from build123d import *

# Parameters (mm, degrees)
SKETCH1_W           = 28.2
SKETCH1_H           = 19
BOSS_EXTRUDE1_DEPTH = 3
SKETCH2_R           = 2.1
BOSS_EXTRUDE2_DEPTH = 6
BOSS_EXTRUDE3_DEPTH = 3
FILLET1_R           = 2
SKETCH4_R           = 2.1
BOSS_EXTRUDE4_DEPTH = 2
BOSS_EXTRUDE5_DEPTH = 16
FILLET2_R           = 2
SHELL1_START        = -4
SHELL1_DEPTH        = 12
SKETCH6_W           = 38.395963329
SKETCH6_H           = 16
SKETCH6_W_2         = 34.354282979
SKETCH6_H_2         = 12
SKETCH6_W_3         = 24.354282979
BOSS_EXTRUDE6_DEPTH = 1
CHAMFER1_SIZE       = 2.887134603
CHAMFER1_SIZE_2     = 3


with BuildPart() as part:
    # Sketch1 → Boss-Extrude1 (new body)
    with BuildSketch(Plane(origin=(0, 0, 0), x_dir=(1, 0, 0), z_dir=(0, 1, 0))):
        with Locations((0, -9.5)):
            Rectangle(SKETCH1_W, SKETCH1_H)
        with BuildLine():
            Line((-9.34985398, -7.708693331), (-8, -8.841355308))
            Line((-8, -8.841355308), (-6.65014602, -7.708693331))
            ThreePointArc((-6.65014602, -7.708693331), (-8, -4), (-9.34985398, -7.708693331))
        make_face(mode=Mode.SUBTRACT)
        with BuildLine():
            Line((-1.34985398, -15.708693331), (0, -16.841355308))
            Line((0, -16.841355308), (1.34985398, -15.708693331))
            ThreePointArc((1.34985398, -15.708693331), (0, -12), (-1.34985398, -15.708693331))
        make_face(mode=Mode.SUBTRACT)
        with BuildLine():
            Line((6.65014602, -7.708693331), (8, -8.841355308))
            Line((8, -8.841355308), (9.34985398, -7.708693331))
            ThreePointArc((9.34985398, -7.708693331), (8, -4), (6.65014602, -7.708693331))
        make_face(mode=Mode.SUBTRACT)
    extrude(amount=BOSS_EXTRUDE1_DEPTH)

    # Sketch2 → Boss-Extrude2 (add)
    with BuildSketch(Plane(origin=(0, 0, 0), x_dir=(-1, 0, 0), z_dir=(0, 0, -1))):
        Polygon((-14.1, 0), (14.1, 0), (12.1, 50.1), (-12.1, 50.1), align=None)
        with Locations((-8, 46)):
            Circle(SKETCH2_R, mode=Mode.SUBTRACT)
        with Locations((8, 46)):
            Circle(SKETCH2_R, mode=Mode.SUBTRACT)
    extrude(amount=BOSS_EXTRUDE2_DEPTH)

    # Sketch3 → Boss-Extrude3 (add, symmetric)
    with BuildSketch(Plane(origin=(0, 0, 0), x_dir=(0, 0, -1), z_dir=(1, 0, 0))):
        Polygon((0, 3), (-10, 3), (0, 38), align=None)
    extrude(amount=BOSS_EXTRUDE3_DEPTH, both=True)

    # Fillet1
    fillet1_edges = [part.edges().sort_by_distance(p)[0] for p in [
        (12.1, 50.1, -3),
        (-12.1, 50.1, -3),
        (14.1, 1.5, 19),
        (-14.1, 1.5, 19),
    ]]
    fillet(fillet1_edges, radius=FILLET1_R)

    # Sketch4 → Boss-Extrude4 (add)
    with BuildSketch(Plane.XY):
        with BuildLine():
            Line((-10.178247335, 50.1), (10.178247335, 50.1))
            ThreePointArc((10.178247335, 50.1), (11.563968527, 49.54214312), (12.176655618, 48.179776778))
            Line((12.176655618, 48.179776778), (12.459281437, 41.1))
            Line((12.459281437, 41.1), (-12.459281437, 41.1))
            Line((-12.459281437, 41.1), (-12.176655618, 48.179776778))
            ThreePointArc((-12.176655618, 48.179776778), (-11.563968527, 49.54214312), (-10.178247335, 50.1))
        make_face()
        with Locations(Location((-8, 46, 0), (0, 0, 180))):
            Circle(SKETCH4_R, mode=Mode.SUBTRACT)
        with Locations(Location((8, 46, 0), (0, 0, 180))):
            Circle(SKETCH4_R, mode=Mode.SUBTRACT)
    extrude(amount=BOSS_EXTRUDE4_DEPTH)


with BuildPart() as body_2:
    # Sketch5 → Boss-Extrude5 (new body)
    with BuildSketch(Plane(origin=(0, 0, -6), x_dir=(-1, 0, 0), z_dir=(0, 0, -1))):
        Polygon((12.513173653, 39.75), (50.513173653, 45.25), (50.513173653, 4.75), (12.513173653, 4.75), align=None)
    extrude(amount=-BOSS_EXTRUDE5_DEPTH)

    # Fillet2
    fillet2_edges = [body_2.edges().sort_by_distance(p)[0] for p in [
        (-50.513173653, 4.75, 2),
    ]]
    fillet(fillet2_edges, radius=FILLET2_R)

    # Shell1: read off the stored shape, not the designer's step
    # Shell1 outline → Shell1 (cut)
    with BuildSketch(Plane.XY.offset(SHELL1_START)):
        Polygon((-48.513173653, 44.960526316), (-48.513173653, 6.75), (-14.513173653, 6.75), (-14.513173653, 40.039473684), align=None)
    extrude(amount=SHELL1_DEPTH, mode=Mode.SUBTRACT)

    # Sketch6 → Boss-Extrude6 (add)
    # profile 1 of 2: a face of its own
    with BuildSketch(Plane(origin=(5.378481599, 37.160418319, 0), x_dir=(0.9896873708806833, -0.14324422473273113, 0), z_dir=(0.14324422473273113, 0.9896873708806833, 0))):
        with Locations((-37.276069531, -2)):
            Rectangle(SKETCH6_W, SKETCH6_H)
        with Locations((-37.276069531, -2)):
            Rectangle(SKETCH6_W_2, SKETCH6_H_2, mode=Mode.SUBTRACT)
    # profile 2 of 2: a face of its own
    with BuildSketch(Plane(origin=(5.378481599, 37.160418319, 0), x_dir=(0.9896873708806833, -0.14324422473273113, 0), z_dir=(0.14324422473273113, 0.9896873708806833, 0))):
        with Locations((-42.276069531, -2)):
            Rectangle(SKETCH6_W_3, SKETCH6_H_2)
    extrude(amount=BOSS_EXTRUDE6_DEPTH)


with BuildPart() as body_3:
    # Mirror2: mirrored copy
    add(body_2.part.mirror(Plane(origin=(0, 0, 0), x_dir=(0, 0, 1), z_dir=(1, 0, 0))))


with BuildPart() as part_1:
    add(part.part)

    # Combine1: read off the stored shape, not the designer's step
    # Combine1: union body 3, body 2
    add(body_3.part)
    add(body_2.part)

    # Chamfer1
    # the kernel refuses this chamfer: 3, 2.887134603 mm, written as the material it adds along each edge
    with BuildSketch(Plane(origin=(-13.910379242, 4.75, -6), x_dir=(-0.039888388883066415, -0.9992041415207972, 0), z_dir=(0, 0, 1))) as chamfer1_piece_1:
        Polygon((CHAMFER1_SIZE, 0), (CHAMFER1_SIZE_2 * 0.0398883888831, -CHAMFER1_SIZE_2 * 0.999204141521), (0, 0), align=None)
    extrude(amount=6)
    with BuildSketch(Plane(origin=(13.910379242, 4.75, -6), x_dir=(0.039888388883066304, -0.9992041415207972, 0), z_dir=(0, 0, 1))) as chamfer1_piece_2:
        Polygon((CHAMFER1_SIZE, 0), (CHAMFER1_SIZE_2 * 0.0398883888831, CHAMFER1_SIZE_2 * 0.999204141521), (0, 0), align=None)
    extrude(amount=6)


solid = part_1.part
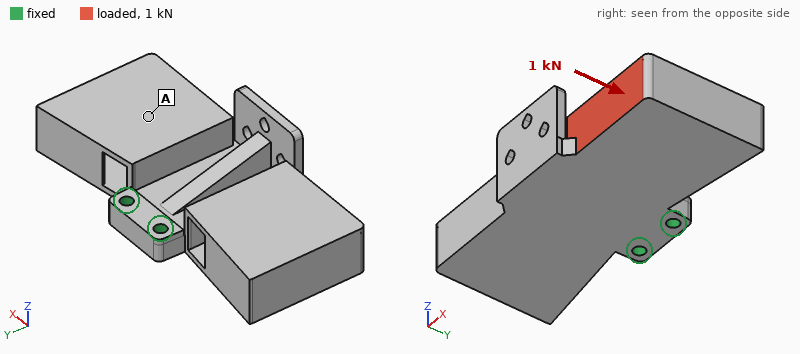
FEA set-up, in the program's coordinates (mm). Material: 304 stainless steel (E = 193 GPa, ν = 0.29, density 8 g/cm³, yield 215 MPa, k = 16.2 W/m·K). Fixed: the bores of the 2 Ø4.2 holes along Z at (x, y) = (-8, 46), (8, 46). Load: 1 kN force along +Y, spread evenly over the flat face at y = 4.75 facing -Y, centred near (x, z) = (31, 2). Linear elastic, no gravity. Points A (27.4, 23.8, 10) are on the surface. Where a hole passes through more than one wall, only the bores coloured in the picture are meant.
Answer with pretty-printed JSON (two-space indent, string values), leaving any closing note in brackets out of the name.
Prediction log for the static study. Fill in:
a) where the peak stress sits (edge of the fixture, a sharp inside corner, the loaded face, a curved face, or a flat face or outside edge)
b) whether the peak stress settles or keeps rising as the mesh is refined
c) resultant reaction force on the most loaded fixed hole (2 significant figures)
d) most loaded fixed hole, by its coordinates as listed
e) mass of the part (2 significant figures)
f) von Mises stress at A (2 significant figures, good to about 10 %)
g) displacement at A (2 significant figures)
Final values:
{
  "where the peak stress sits": "a sharp inside corner",
  "whether the peak stress settles or keeps rising as the mesh is refined": "keeps rising",
  "resultant reaction force on the most loaded fixed hole": "2.3 kN",
  "most loaded fixed hole, by its coordinates as listed": "(8, 46)",
  "mass of the part": "220 g",
  "von Mises stress at A": "9.2 MPa",
  "displacement at A": "27 µm"
}
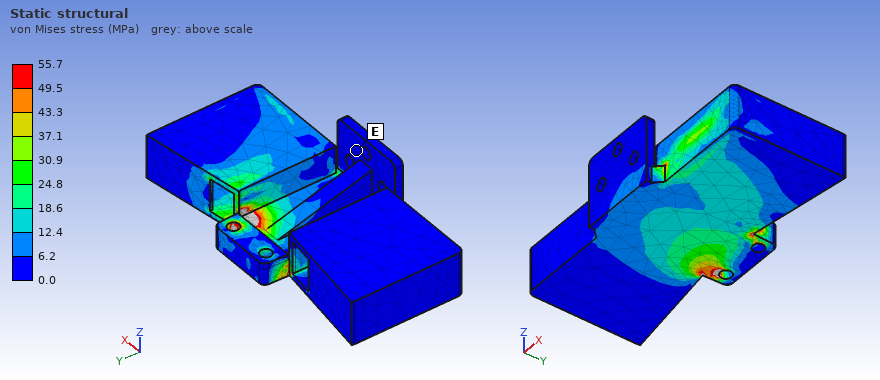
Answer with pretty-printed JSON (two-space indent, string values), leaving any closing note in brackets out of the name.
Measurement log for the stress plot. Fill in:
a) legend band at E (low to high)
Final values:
{
  "legend band at E": "0.0 to 6.2 MPa"
}
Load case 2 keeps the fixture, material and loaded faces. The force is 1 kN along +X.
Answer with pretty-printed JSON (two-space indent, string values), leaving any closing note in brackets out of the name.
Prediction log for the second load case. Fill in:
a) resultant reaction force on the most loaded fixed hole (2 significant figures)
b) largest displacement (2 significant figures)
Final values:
{
  "resultant reaction force on the most loaded fixed hole": "2.3 kN",
  "largest displacement": "65 µm"
}
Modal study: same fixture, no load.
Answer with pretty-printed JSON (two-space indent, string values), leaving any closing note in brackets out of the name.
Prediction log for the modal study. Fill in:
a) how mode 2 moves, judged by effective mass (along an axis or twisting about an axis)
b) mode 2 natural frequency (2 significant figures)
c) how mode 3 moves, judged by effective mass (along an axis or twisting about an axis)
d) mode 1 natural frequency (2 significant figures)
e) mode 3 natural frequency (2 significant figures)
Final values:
{
  "how mode 2 moves, judged by effective mass": "along Z",
  "mode 2 natural frequency": "1200 Hz",
  "how mode 3 moves, judged by effective mass": "twisting about X",
  "mode 1 natural frequency": "1100 Hz",
  "mode 3 natural frequency": "2000 Hz"
}
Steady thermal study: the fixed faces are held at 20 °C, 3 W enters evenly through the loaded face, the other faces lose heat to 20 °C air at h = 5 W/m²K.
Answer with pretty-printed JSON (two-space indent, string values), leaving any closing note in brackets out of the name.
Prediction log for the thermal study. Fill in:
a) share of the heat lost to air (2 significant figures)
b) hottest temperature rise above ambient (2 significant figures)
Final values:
{
  "share of the heat lost to air": "47 %",
  "hottest temperature rise above ambient": "38 K"
}
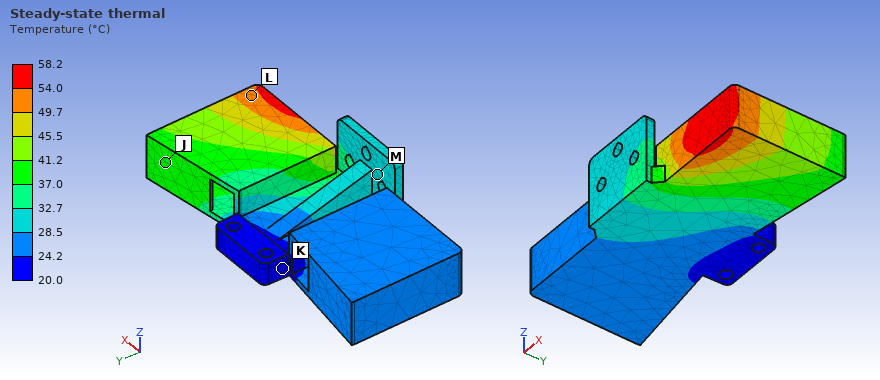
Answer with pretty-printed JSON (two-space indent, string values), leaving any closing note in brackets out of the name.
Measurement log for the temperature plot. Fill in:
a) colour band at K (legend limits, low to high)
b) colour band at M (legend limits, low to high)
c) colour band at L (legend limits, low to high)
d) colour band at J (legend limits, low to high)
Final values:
{
  "colour band at K": "20.0 to 24.2 °C",
  "colour band at M": "28.5 to 32.7 °C",
  "colour band at L": "49.7 to 54.0 °C",
  "colour band at J": "37.0 to 41.2 °C"
}
